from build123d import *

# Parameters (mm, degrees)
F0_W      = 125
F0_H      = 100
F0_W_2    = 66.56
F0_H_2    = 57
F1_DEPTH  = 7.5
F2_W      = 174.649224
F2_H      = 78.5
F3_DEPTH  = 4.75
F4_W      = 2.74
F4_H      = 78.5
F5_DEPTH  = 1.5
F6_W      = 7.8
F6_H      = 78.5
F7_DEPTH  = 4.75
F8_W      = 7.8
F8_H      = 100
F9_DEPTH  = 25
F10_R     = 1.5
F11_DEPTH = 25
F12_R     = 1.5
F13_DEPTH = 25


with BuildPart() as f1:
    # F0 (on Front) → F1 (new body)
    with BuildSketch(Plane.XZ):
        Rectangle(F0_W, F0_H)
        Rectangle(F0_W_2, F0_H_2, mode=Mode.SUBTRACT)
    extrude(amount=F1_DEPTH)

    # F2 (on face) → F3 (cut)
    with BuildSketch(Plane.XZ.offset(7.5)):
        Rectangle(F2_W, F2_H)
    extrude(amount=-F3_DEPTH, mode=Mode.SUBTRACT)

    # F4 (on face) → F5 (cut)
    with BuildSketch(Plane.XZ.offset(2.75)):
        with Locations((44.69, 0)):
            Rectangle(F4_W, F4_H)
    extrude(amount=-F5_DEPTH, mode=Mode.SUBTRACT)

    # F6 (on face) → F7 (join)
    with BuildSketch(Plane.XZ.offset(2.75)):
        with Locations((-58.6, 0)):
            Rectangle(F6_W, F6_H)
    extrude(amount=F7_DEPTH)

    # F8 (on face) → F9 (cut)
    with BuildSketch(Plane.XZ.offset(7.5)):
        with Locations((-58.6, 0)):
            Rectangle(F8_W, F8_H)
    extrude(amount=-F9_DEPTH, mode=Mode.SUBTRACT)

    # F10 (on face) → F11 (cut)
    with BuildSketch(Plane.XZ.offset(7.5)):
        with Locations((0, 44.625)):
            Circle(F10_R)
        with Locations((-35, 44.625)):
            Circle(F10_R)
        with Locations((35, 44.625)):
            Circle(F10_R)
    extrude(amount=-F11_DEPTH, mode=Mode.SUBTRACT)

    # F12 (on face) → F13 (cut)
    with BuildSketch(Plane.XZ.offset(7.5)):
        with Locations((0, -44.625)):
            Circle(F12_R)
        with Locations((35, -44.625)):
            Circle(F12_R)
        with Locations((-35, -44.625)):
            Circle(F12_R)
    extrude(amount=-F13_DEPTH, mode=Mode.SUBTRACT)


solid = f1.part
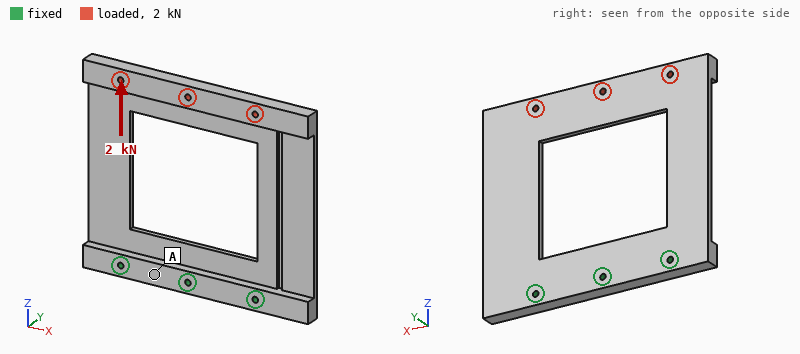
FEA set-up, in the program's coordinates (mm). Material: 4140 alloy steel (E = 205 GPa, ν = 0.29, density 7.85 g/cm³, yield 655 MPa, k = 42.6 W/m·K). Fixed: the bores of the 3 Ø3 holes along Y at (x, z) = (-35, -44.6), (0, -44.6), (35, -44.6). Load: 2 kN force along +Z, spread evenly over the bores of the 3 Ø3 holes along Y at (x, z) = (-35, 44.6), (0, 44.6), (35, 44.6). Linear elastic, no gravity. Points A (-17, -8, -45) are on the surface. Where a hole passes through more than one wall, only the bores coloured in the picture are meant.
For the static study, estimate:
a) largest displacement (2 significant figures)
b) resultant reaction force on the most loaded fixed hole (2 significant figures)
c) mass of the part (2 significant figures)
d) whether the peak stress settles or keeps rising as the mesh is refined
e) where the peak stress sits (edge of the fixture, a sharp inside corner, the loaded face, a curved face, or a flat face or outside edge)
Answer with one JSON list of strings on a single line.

["1.1 mm", "1.2 kN", "260 g", "keeps rising", "a sharp inside corner"]
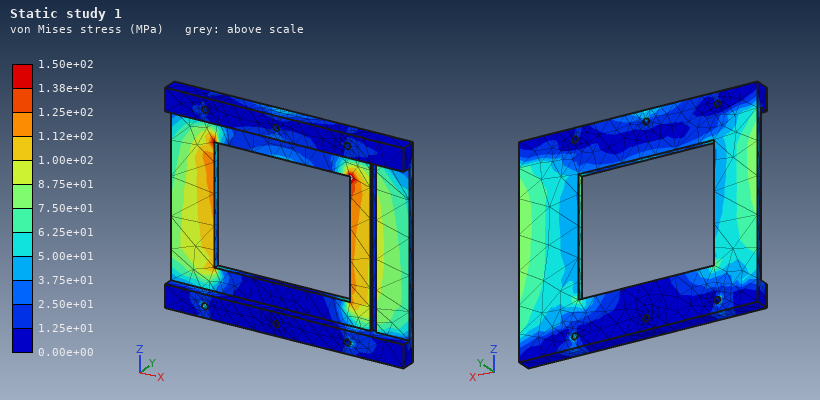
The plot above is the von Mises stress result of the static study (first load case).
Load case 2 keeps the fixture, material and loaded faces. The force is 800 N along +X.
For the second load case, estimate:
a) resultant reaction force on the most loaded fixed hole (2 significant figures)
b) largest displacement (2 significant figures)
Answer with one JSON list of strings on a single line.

["1.0 kN", "0.15 mm"]
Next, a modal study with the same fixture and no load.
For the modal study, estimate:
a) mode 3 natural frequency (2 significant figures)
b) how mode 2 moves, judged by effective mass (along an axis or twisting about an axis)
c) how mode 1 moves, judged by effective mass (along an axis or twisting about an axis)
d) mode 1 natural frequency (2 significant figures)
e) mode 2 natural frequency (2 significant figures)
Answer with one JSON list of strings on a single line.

["1400 Hz", "twisting about Z", "along Y", "150 Hz", "420 Hz"]
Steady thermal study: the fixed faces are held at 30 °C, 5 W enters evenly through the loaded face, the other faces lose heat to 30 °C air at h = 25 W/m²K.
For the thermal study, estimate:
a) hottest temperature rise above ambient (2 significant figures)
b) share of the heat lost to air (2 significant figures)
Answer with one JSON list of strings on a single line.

["22 K", "86 %"]
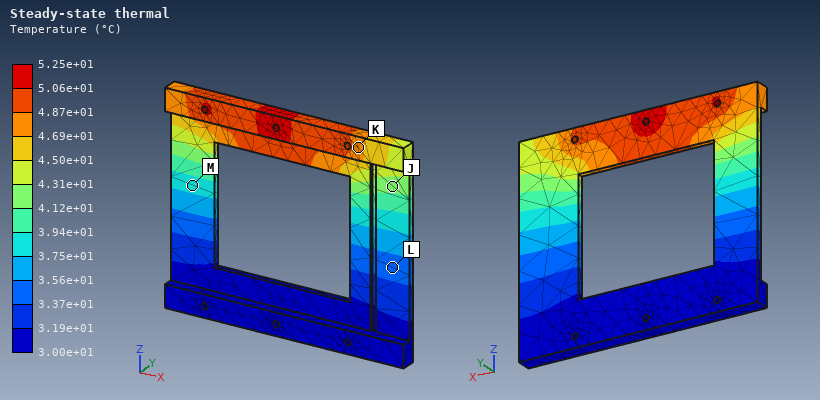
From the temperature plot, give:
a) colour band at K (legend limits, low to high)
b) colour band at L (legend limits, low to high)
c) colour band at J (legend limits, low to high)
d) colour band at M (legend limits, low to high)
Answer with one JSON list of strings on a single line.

["4.69e+01 to 4.87e+01 °C", "3.37e+01 to 3.56e+01 °C", "4.12e+01 to 4.31e+01 °C", "3.75e+01 to 3.94e+01 °C"]
